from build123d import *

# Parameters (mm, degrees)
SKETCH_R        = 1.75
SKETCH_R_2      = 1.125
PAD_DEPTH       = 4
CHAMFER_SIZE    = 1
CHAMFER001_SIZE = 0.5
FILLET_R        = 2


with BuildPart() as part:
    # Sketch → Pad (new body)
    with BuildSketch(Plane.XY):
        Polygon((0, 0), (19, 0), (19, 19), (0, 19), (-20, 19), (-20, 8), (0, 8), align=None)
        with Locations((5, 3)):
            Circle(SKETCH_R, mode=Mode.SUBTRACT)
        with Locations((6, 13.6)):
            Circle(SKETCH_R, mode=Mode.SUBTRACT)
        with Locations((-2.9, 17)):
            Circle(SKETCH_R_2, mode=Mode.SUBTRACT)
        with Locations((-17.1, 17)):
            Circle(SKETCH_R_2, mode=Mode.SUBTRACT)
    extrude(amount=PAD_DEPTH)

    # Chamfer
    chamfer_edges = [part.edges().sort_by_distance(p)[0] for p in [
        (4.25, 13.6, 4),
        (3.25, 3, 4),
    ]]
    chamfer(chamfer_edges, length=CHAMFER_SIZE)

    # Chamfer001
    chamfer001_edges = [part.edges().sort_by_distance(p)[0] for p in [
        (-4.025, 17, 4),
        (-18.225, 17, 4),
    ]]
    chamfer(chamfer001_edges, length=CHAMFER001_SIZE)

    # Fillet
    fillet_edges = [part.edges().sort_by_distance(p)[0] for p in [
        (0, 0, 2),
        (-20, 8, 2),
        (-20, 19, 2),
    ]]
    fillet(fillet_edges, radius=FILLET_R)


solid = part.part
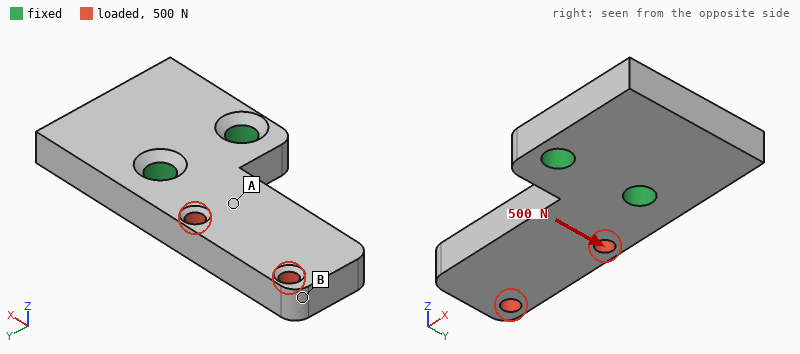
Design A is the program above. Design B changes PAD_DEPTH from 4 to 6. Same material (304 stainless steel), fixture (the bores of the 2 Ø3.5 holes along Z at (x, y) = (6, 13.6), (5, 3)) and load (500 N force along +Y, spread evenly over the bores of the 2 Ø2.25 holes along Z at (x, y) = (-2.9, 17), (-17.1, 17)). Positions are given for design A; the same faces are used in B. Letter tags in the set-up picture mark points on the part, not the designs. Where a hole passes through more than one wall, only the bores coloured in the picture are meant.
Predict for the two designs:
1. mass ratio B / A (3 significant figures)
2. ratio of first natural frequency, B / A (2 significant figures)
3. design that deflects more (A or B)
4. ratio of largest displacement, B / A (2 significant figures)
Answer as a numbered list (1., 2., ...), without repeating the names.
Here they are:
1. 1.50
2. 1.5
3. A
4. 0.65
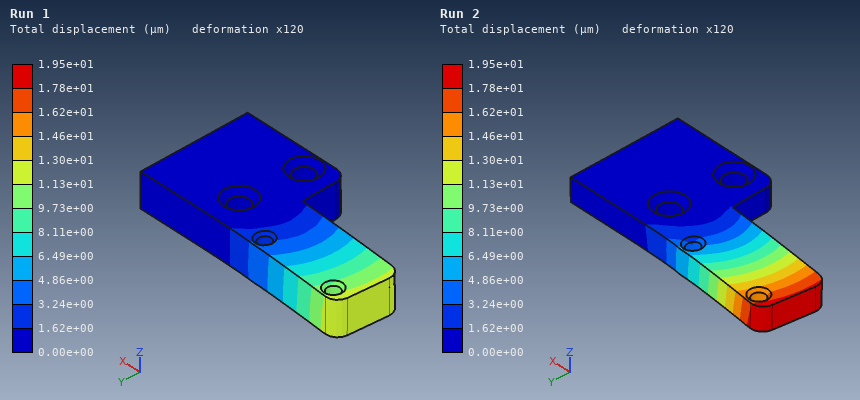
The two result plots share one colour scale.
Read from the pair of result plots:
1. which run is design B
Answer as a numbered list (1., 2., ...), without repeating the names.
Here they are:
1. Run 1
